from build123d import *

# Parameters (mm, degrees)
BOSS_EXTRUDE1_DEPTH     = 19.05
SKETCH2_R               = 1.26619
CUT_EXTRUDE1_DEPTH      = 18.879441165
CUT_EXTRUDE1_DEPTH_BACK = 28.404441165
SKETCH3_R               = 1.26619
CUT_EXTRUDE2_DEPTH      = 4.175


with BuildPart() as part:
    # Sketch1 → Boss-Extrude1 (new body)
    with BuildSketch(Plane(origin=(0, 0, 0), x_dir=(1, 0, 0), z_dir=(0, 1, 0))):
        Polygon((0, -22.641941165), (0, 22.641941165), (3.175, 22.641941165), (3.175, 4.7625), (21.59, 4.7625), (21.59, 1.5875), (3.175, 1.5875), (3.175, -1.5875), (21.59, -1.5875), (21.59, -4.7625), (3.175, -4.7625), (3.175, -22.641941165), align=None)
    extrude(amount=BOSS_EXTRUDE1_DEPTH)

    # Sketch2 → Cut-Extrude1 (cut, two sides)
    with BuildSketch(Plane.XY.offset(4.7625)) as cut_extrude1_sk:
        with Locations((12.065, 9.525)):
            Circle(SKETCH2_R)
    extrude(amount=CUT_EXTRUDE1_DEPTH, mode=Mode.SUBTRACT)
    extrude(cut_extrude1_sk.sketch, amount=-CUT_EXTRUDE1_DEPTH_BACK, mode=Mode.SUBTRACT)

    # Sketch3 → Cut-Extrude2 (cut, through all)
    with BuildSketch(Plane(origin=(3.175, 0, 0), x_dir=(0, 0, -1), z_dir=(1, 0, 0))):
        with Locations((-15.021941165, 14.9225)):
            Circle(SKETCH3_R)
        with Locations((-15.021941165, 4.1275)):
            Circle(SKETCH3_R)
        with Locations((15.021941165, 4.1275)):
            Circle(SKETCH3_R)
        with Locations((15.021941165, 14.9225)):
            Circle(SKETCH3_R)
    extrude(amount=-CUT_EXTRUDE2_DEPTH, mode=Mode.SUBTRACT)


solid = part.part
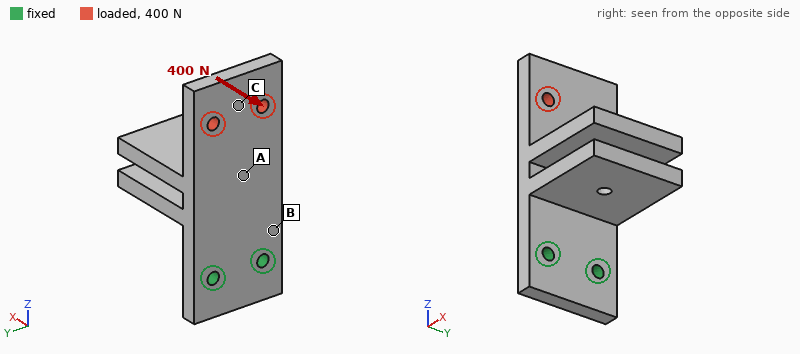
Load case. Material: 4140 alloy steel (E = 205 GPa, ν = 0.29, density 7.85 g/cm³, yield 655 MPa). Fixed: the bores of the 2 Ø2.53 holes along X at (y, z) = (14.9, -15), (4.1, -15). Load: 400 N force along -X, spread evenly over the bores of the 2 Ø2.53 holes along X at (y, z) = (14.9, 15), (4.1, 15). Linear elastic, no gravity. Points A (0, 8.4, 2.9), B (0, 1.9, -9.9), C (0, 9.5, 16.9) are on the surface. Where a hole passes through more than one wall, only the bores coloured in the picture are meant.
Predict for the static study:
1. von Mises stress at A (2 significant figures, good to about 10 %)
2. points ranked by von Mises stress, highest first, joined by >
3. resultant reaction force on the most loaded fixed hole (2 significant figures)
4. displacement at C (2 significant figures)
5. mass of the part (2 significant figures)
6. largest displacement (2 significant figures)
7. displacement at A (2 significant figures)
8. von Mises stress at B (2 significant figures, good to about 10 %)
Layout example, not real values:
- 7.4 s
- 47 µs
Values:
- 120 MPa
- B > A > C
- 200 N
- 0.34 mm
- 38 g
- 0.43 mm
- 0.14 mm
- 310 MPa
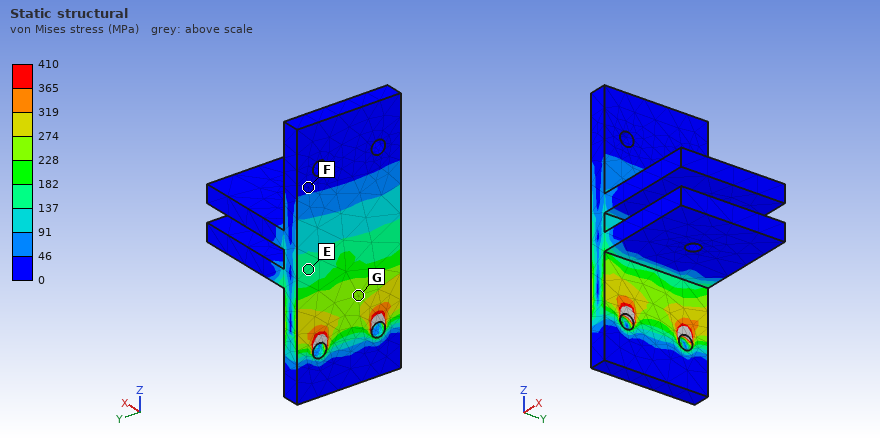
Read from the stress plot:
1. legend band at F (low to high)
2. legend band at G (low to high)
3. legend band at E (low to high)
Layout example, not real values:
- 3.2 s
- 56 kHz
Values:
- 0 to 46 MPa
- 228 to 274 MPa
- 137 to 182 MPa
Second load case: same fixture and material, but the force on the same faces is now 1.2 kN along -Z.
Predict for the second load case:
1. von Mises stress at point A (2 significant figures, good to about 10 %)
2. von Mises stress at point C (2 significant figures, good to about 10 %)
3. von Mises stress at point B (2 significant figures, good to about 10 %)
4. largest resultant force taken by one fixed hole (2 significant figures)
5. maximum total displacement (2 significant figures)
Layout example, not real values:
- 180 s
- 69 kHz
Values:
- 22 MPa
- 8.8 MPa
- 20 MPa
- 600 N
- 4.1 µm
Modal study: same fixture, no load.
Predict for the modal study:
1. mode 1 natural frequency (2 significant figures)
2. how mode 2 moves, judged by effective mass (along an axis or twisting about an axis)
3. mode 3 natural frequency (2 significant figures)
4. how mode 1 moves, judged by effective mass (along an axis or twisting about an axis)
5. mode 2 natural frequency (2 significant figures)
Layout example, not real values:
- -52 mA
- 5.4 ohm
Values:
- 1500 Hz
- along Y
- 5500 Hz
- along X
- 3900 Hz
